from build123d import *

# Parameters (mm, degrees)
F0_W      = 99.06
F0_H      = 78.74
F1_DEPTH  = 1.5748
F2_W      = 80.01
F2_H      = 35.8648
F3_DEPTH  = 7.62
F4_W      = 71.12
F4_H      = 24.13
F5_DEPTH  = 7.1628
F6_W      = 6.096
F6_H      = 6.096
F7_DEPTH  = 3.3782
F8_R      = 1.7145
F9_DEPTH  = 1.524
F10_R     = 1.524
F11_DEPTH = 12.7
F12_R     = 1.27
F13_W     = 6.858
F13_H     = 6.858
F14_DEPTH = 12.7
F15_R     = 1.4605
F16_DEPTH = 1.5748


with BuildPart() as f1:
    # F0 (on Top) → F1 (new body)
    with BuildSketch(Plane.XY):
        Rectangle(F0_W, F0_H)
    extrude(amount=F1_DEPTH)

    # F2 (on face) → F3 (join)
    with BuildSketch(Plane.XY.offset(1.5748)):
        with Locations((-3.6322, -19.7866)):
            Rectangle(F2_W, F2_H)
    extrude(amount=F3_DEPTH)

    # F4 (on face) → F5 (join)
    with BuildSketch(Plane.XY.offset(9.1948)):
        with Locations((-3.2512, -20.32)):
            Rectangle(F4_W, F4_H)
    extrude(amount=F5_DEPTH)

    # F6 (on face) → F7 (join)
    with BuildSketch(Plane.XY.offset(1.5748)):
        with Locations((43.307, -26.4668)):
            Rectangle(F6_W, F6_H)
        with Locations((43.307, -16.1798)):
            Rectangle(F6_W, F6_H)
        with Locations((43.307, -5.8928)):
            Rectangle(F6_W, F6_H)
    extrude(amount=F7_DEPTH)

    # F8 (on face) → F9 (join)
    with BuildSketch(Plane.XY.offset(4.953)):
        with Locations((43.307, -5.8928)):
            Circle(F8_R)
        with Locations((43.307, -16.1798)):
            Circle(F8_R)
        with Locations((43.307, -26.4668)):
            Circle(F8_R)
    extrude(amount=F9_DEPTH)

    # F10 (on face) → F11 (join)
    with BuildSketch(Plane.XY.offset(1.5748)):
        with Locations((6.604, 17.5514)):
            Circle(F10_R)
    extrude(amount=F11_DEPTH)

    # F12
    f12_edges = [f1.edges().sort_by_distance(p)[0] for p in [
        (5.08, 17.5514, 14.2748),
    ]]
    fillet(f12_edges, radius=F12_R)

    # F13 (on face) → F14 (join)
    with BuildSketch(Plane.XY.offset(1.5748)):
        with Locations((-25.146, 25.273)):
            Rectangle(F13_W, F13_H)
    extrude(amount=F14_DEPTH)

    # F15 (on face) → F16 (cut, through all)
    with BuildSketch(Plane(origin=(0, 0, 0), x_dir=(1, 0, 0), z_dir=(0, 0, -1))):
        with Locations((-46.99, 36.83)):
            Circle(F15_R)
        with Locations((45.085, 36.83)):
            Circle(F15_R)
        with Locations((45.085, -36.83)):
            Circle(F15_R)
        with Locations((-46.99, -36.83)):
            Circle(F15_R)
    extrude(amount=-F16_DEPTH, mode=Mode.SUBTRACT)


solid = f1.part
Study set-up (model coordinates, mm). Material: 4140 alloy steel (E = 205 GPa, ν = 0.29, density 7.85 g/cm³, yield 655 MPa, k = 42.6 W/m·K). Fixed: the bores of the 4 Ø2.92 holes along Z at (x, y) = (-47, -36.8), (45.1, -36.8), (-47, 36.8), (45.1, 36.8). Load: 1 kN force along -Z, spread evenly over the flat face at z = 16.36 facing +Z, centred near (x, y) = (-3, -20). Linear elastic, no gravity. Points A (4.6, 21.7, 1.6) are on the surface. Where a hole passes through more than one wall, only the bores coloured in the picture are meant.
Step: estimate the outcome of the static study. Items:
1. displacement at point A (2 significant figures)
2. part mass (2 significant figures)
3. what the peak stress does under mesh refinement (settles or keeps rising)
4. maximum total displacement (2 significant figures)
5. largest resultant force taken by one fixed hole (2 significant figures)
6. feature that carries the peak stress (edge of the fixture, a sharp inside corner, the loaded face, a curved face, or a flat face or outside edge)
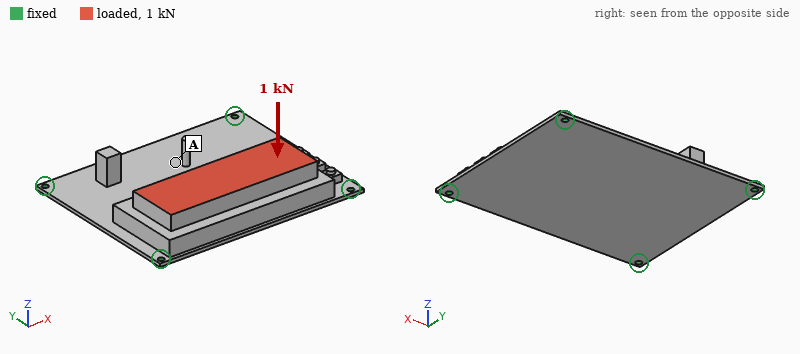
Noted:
0.19 mm
370 g
keeps rising
0.22 mm
530 N
edge of the fixture
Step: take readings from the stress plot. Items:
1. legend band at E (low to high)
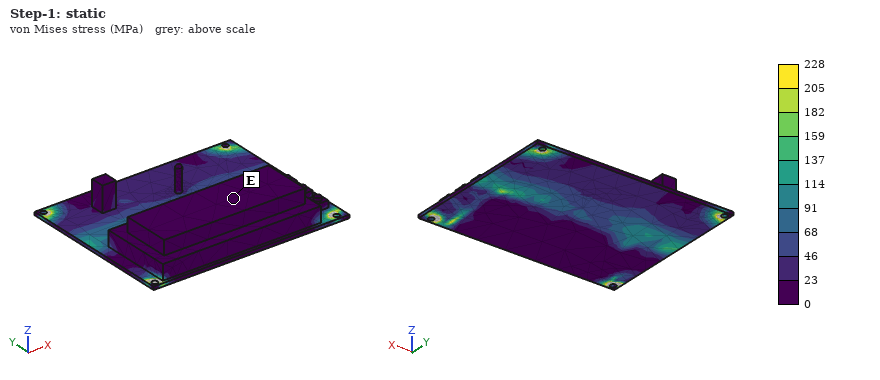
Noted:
0 to 23 MPa
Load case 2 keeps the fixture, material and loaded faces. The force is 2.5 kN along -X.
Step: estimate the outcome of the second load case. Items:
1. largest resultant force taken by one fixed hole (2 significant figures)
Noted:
1.2 kN
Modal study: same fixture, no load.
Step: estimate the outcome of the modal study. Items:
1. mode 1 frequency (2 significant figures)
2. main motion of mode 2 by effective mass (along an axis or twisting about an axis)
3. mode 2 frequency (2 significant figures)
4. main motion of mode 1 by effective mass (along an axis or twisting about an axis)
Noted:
630 Hz
twisting about X
1500 Hz
along Z
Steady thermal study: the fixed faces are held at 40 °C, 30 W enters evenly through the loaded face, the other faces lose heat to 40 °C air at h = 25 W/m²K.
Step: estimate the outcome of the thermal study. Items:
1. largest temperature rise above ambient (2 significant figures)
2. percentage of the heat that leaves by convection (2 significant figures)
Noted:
61 K
59 %
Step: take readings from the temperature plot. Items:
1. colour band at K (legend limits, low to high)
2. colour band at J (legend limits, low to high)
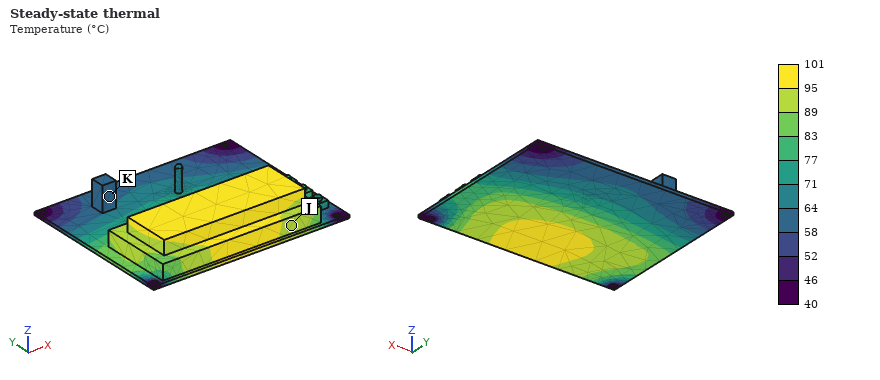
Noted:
58 to 64 °C
89 to 95 °C
